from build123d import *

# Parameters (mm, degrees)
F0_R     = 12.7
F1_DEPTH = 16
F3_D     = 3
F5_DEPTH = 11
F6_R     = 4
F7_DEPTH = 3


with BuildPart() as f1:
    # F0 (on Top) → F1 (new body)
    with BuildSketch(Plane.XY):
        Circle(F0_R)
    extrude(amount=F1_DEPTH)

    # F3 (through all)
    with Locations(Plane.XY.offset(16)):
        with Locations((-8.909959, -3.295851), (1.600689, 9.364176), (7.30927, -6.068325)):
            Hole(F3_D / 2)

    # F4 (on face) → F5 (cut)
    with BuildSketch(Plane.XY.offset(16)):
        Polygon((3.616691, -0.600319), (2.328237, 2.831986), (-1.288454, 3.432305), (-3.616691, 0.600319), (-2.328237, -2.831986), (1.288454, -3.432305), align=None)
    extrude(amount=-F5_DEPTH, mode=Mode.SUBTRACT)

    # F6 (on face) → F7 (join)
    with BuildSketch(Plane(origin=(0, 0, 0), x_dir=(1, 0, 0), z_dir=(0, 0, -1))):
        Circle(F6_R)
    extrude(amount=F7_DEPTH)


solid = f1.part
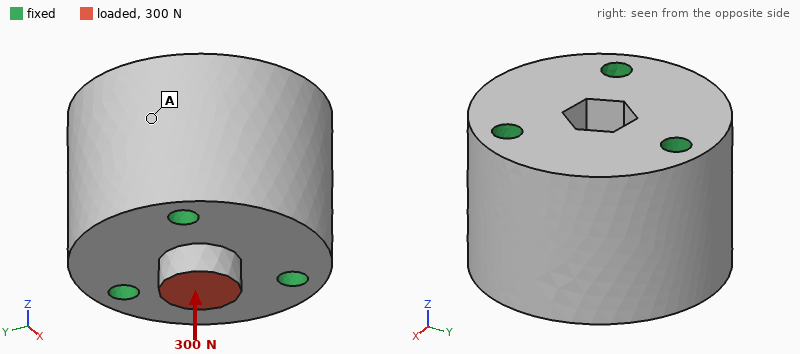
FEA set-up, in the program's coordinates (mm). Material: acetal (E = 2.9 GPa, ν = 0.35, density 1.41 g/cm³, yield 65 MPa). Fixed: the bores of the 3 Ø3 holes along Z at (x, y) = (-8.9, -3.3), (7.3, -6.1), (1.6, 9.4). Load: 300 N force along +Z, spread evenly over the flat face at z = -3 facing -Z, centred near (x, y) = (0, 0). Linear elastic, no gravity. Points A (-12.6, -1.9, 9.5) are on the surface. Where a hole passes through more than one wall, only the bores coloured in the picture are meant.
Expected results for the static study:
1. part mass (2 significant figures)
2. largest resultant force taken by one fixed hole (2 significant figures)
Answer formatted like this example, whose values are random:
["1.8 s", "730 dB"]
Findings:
["11 g", "110 N"]
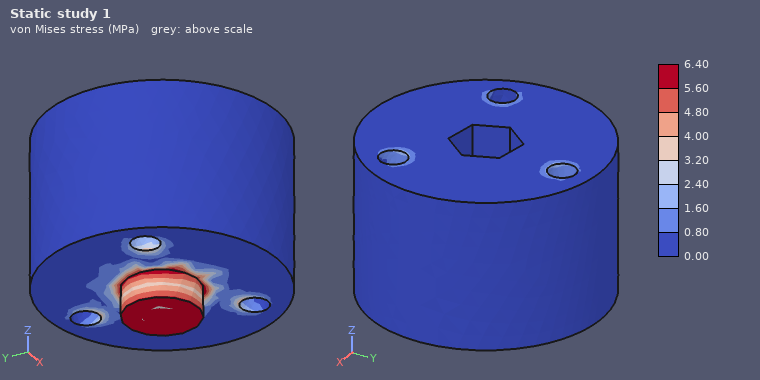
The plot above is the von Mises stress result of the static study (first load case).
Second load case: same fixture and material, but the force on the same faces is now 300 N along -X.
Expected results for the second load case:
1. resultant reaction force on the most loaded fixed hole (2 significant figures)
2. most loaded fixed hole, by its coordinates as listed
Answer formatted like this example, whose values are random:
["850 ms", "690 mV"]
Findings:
["170 N", "(-8.9, -3.3)"]
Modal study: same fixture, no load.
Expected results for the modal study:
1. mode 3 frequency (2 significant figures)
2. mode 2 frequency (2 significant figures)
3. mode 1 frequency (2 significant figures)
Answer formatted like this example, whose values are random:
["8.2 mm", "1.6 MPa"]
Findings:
["20 kHz", "20 kHz", "20 kHz"]
